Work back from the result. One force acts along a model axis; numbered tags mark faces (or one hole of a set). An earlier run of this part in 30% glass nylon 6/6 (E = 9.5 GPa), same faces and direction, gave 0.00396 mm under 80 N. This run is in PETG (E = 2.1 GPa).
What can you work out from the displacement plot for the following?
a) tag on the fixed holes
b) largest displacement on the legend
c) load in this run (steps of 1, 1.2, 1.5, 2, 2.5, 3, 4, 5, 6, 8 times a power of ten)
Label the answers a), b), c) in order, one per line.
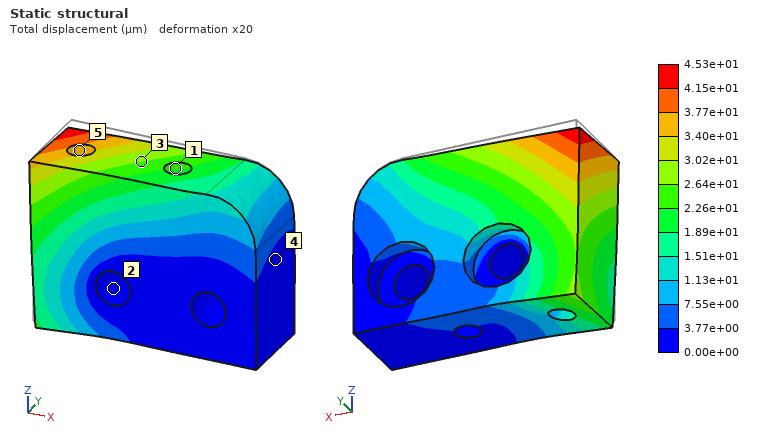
a) 2
b) 4.53e+01 µm
c) 200 N
